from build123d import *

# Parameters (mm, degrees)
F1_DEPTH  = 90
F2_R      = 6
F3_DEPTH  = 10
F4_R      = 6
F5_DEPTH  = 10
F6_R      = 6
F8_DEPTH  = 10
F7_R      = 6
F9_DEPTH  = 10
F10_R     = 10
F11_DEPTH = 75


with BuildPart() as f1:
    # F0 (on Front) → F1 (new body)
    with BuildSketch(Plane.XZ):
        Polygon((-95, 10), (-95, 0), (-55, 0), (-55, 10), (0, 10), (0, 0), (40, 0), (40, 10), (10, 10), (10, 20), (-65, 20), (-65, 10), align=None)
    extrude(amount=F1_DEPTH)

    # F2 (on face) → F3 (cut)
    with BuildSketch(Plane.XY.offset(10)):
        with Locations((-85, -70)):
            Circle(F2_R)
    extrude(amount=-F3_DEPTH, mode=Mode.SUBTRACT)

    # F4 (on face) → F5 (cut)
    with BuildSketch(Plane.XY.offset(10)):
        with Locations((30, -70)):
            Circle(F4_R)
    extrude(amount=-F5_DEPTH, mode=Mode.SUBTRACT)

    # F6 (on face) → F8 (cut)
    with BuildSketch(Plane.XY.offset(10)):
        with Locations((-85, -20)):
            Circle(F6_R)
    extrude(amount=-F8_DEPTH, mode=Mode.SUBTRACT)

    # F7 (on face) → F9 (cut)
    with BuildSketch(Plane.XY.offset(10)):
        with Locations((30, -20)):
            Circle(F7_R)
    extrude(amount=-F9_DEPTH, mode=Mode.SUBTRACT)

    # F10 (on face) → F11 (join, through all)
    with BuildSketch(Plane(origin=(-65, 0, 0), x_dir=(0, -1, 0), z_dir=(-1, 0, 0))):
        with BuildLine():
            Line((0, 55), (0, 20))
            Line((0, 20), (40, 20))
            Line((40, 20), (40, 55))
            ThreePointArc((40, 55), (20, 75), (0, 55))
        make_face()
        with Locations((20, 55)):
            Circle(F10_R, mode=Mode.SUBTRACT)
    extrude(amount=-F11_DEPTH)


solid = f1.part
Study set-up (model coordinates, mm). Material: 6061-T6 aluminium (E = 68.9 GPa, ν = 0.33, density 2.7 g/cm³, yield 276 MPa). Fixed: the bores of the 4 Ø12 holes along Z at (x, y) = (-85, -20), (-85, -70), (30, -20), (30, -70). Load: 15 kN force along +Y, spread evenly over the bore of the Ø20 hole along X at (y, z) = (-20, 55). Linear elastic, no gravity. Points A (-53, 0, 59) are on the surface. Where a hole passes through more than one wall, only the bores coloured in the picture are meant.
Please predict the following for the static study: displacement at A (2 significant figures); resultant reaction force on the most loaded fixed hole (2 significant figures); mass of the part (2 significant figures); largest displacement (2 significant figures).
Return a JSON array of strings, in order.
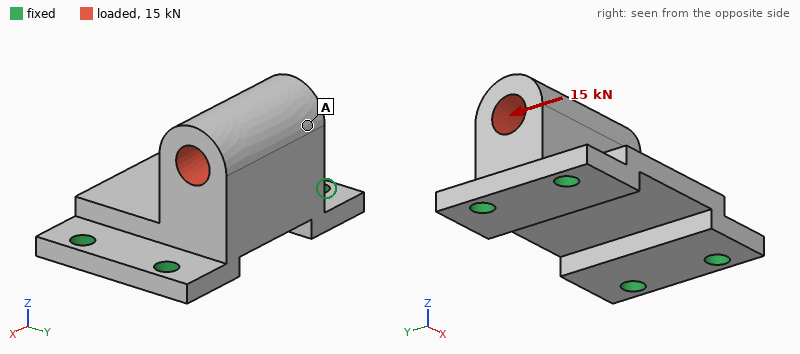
["0.29 mm", "12 kN", "710 g", "0.34 mm"]
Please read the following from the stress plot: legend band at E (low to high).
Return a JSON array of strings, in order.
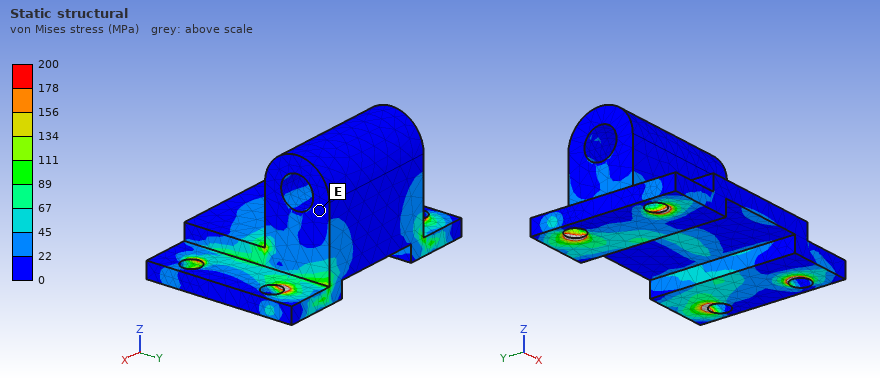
["0 to 22 MPa"]
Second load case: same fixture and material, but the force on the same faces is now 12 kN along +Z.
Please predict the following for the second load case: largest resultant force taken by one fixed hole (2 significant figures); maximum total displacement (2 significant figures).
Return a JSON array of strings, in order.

["7.2 kN", "77 µm"]
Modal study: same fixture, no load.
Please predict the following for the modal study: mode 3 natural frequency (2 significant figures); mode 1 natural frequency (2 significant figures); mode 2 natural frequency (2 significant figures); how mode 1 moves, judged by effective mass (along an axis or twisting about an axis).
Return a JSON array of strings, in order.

["4200 Hz", "2300 Hz", "4200 Hz", "along Y"]
